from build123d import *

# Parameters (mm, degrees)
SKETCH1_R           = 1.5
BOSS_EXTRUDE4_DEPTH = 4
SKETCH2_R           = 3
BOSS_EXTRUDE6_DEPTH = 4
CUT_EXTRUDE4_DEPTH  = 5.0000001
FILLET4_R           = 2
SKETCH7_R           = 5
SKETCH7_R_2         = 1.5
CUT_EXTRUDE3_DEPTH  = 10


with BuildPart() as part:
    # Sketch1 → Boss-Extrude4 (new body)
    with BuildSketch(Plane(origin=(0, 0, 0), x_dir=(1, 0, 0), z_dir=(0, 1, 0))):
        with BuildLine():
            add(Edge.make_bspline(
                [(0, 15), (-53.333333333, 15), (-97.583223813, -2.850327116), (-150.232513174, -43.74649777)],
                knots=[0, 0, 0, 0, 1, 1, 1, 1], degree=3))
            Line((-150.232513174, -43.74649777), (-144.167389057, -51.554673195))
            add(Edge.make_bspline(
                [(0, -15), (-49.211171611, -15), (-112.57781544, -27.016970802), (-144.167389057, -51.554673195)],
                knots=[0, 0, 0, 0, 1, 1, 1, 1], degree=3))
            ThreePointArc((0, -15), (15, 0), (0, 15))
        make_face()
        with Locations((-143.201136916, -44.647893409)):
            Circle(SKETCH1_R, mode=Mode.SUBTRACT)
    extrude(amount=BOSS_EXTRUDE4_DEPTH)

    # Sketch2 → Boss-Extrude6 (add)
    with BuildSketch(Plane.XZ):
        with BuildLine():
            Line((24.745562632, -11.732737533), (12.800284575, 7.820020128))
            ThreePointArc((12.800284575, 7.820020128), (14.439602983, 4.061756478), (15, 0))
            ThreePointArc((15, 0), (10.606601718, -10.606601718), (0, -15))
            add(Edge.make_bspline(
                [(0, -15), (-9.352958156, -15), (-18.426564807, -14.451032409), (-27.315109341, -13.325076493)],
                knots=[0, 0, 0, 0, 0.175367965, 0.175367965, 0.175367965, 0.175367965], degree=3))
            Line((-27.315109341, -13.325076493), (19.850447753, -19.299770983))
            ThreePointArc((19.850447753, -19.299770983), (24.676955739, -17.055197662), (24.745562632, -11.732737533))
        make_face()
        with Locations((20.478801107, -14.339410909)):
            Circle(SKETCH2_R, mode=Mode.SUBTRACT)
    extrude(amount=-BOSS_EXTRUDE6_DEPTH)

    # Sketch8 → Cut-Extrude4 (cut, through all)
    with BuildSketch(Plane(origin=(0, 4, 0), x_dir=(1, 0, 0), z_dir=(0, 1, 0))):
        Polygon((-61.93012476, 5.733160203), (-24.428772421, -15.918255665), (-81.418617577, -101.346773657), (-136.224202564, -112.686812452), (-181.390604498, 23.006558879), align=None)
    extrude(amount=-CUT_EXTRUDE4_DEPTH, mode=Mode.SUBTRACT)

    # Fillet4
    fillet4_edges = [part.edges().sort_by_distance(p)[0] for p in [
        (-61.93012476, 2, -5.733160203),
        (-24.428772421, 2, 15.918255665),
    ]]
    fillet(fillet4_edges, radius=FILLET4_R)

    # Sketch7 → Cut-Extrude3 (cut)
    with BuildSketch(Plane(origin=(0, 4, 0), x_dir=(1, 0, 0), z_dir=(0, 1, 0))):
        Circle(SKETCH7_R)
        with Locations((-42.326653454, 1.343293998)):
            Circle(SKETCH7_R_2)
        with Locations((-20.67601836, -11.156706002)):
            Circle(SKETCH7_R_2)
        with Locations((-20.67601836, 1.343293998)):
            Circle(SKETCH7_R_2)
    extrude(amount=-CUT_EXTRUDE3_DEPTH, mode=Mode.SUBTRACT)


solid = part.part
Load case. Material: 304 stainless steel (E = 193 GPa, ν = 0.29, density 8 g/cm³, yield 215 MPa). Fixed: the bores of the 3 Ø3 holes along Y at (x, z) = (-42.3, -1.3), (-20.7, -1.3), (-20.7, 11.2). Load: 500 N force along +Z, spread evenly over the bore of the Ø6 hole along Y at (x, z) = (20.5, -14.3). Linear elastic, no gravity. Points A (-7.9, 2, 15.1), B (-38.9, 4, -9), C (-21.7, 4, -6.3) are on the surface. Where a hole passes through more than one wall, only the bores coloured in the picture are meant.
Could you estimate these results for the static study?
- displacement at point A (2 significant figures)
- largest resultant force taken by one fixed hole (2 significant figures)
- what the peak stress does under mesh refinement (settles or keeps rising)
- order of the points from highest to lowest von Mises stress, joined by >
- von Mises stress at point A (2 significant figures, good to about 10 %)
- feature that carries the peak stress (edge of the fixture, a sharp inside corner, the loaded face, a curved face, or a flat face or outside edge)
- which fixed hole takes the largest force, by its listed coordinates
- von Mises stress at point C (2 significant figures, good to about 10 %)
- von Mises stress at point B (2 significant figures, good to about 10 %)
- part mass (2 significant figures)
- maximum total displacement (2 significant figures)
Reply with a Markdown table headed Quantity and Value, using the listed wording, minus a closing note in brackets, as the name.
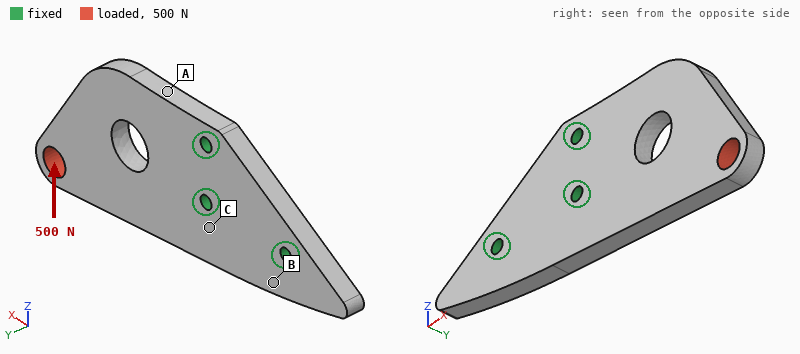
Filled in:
| Quantity | Value |
|---|---|
| displacement at point A | 4.0 µm |
| largest resultant force taken by one fixed hole | 1.1 kN |
| what the peak stress does under mesh refinement | keeps rising |
| order of the points from highest to lowest von Mises stress, joined by > | A > C > B |
| von Mises stress at point A | 32 MPa |
| feature that carries the peak stress | edge of the fixture |
| which fixed hole takes the largest force, by its listed coordinates | (-20.7, 11.2) |
| von Mises stress at point C | 16 MPa |
| von Mises stress at point B | 7.5 MPa |
| part mass | 57 g |
| maximum total displacement | 20 µm |
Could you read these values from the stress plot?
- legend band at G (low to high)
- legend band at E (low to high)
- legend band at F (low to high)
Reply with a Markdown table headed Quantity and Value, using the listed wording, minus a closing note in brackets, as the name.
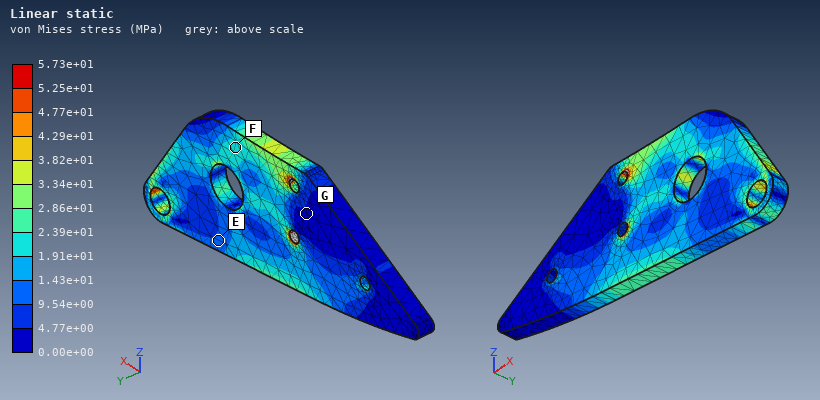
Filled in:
| Quantity | Value |
|---|---|
| legend band at G | 0.00e+00 to 4.77e+00 MPa |
| legend band at E | 9.54e+00 to 1.43e+01 MPa |
| legend band at F | 1.91e+01 to 2.39e+01 MPa |
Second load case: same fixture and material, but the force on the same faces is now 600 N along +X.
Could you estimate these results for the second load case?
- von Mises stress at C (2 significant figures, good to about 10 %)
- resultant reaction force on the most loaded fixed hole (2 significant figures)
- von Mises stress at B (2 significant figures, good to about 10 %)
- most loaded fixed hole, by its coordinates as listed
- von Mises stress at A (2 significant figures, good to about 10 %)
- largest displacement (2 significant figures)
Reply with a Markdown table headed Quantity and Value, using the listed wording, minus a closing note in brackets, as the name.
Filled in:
| Quantity | Value |
|---|---|
| von Mises stress at C | 11 MPa |
| resultant reaction force on the most loaded fixed hole | 660 N |
| von Mises stress at B | 4.9 MPa |
| most loaded fixed hole, by its coordinates as listed | (-20.7, -1.3) |
| von Mises stress at A | 9.9 MPa |
| largest displacement | 11 µm |
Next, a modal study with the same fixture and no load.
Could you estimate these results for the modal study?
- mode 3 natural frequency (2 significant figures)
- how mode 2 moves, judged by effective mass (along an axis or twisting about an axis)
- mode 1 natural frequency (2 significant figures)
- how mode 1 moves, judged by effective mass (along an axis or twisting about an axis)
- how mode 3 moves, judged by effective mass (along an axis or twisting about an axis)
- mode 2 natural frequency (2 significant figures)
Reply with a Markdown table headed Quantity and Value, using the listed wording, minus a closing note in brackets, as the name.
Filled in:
| Quantity | Value |
|---|---|
| mode 3 natural frequency | 8800 Hz |
| how mode 2 moves, judged by effective mass | twisting about X |
| mode 1 natural frequency | 1800 Hz |
| how mode 1 moves, judged by effective mass | along Y |
| how mode 3 moves, judged by effective mass | along Z |
| mode 2 natural frequency | 5600 Hz |
